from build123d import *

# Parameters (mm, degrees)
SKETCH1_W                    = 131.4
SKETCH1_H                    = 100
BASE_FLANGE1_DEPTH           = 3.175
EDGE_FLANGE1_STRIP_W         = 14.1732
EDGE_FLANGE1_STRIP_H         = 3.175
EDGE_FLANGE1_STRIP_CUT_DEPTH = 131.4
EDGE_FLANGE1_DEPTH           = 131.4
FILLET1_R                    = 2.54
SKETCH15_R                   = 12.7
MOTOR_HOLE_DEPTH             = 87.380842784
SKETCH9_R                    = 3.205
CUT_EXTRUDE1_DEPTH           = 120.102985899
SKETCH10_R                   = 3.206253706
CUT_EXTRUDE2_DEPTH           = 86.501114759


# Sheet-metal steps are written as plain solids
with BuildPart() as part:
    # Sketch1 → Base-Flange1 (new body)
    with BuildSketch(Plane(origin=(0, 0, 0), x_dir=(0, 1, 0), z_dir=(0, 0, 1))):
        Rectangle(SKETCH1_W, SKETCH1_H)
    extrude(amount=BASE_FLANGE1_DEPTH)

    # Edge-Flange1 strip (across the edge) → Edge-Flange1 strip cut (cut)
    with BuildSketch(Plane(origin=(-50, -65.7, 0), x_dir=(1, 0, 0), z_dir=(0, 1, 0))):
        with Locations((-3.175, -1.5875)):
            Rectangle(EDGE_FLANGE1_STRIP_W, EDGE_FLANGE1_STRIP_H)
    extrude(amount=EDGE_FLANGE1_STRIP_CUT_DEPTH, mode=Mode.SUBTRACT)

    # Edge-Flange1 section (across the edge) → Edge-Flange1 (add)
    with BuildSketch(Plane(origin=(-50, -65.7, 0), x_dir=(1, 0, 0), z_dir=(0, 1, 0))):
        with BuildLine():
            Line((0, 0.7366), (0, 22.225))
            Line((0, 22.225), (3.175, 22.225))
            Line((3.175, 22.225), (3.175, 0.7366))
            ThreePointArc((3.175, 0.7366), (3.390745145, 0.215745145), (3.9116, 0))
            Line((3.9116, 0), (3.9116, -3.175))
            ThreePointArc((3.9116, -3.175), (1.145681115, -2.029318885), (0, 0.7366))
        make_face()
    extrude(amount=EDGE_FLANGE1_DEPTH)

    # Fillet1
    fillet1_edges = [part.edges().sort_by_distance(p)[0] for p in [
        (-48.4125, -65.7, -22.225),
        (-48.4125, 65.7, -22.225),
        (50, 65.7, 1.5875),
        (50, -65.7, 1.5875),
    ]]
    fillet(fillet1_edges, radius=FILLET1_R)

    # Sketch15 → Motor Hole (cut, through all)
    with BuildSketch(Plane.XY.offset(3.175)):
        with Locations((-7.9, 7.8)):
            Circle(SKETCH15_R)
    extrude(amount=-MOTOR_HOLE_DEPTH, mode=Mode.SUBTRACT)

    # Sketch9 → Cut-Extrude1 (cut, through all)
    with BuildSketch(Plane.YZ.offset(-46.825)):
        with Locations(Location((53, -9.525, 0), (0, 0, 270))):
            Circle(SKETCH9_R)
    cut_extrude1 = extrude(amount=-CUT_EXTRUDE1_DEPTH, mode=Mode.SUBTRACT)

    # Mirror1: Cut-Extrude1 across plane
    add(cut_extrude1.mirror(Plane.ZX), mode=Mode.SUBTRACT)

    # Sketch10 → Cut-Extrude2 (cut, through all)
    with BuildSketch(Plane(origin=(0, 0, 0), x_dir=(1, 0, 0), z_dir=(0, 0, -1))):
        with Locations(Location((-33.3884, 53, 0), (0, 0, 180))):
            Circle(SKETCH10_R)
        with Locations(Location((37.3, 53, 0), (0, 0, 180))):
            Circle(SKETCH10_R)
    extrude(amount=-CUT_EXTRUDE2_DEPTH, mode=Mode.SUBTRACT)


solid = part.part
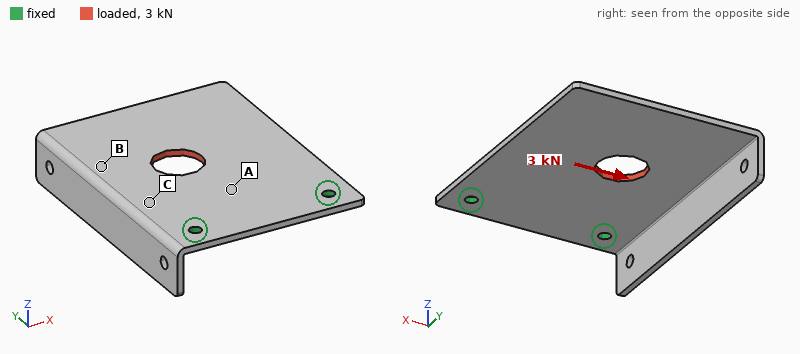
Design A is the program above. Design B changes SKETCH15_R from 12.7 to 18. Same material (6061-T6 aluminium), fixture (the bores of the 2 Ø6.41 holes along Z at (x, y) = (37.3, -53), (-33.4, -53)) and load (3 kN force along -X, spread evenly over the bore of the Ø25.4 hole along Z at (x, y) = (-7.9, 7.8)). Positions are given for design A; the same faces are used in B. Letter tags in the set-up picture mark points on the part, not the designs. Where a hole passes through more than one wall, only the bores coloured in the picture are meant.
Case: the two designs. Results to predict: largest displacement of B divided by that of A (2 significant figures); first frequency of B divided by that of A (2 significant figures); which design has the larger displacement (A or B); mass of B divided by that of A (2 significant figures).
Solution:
1.2
1.0
B
0.97
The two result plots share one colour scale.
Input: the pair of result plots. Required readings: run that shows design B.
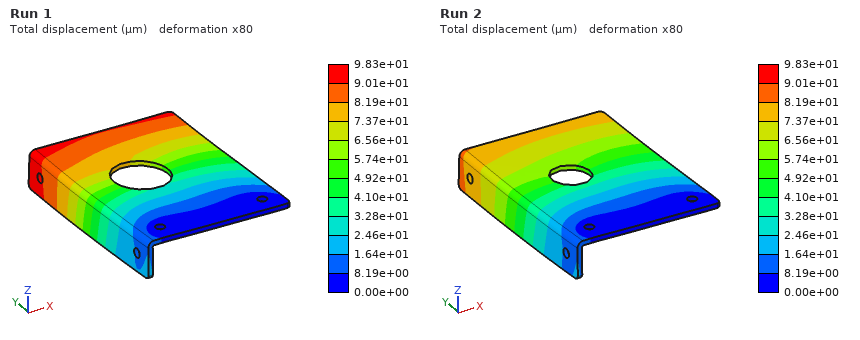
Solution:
Run 1
